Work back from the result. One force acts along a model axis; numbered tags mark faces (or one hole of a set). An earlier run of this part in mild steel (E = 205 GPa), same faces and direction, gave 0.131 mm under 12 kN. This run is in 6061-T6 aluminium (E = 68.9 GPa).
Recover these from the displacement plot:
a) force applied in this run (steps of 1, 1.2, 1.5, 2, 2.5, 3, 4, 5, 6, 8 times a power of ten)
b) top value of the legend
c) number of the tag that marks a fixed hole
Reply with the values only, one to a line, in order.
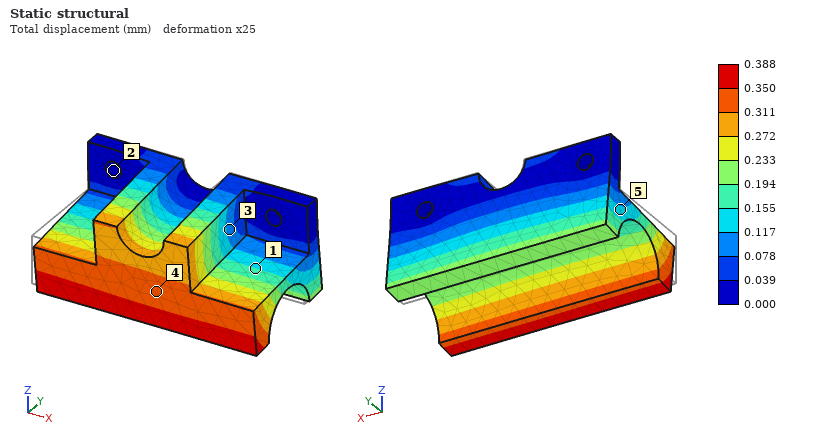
12 kN
0.388 mm
2
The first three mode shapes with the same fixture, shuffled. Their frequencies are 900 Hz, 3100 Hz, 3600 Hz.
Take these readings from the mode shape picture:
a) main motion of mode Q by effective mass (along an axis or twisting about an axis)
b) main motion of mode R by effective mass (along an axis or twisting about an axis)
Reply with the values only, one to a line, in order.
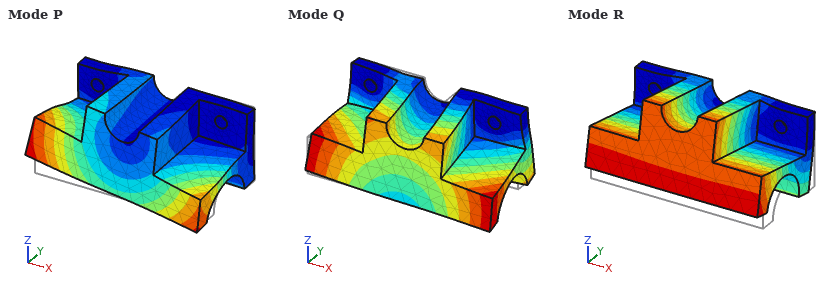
along X
along Z
